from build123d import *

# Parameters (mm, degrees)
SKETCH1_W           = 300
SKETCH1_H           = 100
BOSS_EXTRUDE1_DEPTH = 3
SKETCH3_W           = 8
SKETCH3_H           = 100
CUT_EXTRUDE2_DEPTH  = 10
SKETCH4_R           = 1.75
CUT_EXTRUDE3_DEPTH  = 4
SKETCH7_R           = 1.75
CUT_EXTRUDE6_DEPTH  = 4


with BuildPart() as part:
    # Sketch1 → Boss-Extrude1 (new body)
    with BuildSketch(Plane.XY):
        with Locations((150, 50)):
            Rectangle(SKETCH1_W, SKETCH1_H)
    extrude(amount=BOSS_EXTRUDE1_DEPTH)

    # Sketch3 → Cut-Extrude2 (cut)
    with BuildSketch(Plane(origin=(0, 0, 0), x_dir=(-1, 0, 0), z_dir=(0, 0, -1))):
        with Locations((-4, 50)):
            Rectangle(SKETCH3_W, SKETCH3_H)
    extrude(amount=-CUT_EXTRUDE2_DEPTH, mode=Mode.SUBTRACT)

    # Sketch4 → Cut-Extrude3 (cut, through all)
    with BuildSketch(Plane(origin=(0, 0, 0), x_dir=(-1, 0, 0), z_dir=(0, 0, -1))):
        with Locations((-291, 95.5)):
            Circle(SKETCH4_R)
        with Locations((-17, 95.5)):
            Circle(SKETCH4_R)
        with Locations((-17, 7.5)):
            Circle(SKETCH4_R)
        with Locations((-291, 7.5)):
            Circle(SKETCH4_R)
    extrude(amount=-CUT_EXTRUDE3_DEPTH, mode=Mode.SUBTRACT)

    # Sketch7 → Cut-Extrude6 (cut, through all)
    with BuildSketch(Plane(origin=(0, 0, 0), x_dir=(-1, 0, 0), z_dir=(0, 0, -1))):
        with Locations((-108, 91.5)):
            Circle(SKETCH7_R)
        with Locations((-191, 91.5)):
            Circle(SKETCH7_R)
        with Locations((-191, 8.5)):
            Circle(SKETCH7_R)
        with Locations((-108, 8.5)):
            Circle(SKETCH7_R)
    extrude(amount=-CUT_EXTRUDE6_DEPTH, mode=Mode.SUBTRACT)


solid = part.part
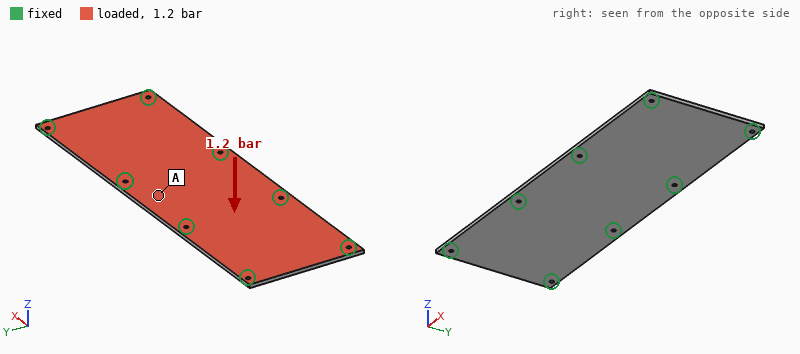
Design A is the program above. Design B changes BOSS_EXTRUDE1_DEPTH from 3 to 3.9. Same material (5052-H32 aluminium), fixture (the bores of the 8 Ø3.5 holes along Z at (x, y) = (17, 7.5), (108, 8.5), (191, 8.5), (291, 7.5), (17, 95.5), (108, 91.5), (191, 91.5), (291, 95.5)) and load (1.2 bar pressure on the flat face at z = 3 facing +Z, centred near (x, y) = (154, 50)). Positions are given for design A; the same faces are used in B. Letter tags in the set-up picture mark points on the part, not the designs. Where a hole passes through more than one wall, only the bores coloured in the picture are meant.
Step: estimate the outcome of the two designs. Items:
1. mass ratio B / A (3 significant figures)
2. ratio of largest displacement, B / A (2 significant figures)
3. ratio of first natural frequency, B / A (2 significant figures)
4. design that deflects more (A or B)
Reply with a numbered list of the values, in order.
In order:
1. 1.30
2. 0.47
3. 1.3
4. A
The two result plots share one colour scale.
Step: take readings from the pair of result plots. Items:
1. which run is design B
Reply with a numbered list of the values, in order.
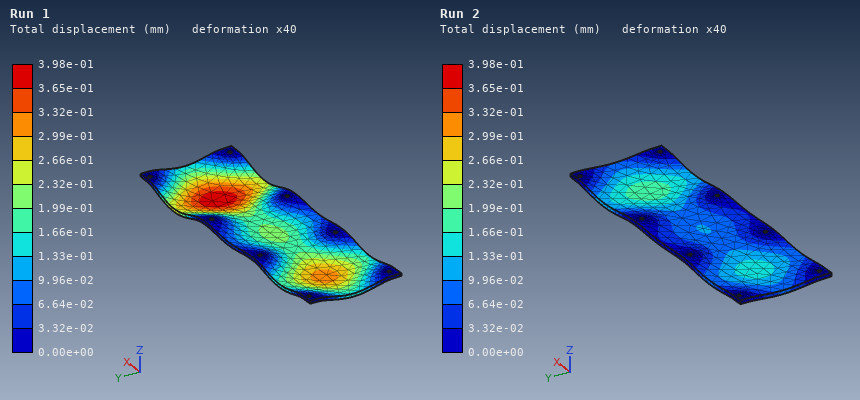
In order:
1. Run 2
